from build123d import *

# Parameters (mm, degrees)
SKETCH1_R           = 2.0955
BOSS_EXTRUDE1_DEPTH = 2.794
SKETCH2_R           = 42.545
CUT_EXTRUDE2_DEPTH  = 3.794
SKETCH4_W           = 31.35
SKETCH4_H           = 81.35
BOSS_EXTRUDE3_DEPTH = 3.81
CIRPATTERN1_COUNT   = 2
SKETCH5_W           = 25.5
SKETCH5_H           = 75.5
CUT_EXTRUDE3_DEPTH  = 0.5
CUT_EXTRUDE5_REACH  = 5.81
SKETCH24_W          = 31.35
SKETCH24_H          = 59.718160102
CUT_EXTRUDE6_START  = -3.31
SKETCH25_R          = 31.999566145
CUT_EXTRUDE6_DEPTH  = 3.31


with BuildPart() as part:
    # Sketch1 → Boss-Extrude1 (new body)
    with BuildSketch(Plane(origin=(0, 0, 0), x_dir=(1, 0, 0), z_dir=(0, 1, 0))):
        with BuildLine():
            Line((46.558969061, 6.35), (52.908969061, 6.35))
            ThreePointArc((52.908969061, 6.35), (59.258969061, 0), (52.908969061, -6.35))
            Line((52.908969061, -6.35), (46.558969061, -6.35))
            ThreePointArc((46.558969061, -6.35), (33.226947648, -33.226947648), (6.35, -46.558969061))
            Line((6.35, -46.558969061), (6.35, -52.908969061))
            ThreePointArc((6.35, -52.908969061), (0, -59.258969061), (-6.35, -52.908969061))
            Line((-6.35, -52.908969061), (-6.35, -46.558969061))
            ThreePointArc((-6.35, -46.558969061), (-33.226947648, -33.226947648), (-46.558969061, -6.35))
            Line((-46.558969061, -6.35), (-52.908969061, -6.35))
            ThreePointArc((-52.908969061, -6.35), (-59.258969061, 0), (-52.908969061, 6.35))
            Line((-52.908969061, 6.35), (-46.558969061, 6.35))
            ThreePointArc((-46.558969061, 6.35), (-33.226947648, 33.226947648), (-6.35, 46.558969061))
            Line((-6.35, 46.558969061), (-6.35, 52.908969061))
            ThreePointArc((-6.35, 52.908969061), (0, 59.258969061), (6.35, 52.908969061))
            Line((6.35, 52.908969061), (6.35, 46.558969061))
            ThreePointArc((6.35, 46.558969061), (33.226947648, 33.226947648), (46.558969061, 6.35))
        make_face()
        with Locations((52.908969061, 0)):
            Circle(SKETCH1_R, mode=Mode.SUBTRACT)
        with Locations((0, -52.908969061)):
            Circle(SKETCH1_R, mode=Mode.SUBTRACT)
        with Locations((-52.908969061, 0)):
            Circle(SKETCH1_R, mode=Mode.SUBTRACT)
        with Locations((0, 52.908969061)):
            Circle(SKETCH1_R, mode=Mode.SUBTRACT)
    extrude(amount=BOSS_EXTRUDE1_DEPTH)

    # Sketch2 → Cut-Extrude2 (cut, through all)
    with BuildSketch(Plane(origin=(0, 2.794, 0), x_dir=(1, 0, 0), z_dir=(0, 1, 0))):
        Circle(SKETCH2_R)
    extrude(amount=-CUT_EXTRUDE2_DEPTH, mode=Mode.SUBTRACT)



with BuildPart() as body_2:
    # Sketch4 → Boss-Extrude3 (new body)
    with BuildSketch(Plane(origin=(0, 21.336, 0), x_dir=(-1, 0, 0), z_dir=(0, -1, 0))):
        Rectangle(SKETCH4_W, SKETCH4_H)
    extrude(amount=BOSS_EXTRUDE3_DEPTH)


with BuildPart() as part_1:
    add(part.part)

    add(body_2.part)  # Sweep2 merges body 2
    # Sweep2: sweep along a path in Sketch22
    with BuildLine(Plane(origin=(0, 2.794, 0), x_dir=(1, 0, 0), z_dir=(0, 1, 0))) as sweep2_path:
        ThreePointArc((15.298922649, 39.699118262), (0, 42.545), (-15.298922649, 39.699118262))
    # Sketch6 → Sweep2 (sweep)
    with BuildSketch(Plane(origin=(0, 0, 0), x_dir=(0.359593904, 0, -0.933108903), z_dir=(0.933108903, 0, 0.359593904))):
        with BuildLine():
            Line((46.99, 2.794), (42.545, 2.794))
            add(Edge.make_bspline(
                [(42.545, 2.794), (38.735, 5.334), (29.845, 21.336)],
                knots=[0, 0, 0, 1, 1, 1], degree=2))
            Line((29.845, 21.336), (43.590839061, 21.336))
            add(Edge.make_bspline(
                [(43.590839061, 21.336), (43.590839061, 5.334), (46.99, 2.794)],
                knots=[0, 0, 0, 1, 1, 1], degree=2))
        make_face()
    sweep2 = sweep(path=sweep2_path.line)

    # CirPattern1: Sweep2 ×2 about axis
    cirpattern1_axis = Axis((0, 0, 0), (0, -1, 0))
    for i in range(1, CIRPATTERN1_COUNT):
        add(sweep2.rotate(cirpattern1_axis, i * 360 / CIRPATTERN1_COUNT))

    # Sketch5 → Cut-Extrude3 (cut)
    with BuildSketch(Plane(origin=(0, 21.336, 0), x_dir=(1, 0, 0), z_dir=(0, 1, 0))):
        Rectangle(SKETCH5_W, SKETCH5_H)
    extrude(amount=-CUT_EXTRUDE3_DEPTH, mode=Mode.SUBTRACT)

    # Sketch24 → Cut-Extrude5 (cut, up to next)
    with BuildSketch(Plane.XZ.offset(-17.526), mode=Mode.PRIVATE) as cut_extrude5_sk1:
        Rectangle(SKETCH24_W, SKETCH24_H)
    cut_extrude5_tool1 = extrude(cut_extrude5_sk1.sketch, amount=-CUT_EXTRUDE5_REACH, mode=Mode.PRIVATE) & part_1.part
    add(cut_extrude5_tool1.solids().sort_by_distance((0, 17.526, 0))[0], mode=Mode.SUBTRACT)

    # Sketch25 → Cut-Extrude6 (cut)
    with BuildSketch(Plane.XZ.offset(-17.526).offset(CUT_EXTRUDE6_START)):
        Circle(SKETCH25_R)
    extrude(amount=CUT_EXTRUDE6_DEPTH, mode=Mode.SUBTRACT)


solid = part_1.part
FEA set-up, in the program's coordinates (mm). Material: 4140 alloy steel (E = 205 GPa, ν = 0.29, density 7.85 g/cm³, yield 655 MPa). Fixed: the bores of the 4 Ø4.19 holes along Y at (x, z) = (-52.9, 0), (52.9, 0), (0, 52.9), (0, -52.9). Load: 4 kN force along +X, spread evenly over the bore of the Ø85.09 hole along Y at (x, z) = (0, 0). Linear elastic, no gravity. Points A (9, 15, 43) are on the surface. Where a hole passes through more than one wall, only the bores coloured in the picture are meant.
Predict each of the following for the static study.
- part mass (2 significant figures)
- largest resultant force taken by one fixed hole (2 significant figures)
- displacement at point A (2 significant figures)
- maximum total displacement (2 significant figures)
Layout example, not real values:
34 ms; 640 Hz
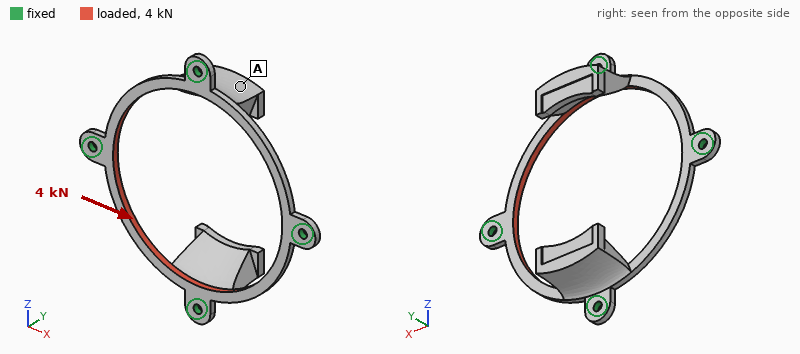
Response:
110 g; 1.6 kN; 12 µm; 24 µm
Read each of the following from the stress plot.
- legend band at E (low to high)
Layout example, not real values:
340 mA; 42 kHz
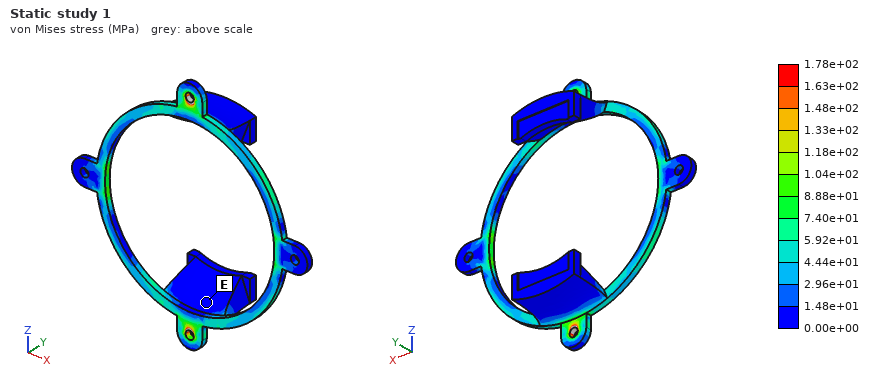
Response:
0.00e+00 to 1.48e+01 MPa
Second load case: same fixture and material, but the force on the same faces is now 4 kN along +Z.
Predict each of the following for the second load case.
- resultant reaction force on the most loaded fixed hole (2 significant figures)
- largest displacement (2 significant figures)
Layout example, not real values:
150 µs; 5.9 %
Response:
1.4 kN; 22 µm
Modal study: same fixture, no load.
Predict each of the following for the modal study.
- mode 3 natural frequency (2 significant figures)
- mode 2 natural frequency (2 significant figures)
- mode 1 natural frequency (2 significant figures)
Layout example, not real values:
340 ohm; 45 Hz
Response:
2000 Hz; 1500 Hz; 1500 Hz
